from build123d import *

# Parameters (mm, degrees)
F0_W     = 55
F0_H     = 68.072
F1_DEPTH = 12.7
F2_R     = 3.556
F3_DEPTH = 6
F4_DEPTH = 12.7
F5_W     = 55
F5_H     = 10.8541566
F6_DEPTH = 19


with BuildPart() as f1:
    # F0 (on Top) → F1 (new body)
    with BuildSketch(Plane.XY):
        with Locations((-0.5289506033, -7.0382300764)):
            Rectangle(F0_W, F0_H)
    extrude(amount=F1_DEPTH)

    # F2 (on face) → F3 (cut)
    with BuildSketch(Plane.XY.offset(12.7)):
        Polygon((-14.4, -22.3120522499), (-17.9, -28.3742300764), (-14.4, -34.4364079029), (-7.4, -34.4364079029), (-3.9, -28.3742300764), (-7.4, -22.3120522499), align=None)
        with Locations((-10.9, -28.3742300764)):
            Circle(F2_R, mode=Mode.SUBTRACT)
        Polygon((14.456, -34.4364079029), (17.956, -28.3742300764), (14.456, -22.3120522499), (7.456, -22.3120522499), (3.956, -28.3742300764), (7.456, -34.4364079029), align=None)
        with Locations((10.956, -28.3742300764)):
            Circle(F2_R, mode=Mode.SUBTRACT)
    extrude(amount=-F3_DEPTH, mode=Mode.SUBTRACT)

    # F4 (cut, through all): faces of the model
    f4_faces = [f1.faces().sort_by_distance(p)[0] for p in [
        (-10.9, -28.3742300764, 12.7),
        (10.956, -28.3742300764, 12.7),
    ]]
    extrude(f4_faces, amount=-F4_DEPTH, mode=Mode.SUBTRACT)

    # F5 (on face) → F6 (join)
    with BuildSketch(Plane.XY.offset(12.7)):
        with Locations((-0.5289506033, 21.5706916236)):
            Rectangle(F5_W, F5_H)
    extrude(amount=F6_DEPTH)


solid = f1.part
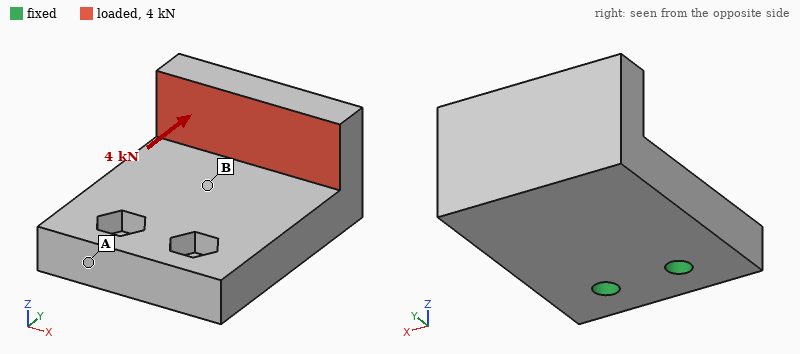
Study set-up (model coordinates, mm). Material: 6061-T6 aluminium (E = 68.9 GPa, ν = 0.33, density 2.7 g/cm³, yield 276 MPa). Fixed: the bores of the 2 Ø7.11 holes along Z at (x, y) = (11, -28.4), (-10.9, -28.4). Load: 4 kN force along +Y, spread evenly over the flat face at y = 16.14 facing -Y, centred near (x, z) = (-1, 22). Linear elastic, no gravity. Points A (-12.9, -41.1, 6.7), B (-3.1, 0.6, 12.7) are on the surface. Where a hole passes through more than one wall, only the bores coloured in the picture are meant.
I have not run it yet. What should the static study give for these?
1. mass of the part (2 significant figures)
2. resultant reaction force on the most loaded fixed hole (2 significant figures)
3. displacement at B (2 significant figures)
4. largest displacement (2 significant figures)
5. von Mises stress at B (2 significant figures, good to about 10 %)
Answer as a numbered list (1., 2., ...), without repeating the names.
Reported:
1. 150 g
2. 2.1 kN
3. 0.11 mm
4. 0.33 mm
5. 46 MPa
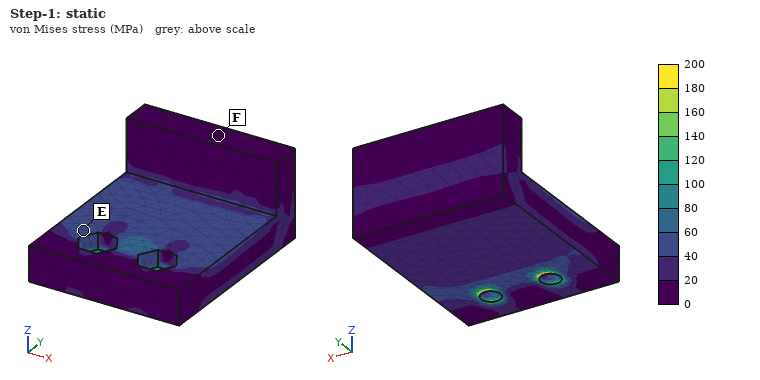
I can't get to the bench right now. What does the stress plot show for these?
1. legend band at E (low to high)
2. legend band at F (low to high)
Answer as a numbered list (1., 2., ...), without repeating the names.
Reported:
1. 40 to 60 MPa
2. 0 to 20 MPa
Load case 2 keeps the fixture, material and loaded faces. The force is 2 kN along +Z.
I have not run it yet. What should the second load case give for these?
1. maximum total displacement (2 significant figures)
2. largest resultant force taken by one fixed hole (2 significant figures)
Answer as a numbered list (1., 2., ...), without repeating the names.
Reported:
1. 0.28 mm
2. 1.1 kN
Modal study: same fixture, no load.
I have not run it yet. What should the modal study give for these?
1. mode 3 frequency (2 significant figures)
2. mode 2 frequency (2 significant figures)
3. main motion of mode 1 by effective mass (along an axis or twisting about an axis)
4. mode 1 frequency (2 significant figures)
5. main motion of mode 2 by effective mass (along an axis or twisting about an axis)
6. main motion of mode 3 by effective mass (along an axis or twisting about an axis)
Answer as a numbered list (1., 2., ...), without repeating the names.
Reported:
1. 5100 Hz
2. 3900 Hz
3. along Z
4. 1600 Hz
5. along X
6. along X
